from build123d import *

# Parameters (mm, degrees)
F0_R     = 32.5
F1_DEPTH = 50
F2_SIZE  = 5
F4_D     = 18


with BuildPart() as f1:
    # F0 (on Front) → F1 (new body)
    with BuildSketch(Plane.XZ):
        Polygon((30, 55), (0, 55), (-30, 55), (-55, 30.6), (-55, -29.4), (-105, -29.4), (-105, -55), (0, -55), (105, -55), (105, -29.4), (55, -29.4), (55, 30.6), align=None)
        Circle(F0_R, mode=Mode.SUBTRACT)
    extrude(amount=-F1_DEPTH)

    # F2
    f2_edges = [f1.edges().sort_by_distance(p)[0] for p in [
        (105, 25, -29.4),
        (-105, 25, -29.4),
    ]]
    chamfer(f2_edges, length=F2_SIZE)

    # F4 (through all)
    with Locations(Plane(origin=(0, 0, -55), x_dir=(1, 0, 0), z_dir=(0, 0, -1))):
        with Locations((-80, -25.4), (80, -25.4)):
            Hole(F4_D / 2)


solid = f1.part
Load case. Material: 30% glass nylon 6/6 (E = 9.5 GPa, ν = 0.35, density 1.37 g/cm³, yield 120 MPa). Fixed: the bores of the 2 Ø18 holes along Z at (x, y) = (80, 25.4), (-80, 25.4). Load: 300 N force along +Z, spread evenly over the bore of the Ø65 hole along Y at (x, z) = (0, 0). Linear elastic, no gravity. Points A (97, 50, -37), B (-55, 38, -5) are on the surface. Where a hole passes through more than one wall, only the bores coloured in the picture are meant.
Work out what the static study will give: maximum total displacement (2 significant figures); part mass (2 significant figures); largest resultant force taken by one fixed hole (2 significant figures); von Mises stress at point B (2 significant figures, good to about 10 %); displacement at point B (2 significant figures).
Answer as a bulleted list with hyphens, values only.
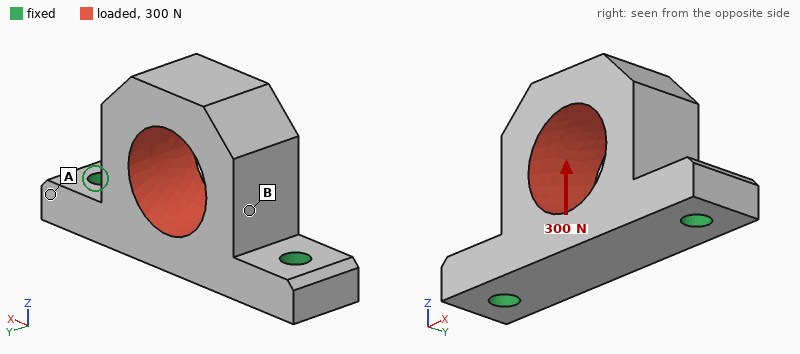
- 3.8 µm
- 720 g
- 150 N
- 0.20 MPa
- 2.6 µm
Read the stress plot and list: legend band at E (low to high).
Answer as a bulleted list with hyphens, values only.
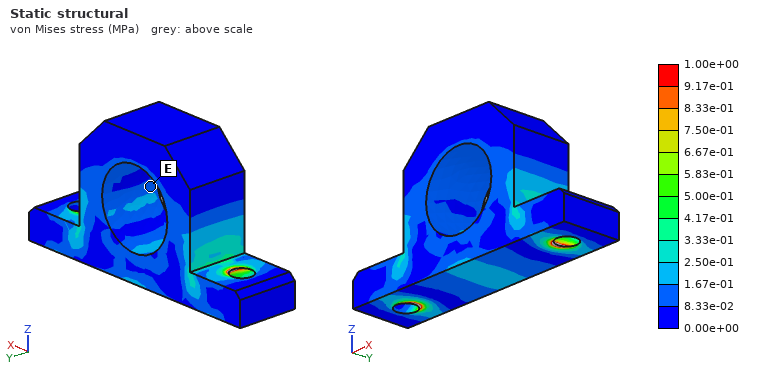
- 8.33e-02 to 1.67e-01 MPa
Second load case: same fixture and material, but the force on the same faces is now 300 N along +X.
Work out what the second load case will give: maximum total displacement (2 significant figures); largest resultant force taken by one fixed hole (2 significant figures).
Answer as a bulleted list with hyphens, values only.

- 5.4 µm
- 180 N
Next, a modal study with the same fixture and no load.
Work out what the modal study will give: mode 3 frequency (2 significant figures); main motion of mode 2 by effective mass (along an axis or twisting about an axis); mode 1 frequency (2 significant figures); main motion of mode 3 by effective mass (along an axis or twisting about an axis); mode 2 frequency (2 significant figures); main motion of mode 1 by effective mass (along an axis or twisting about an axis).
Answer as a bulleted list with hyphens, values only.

- 2200 Hz
- along X
- 800 Hz
- along Z
- 1800 Hz
- along Y
